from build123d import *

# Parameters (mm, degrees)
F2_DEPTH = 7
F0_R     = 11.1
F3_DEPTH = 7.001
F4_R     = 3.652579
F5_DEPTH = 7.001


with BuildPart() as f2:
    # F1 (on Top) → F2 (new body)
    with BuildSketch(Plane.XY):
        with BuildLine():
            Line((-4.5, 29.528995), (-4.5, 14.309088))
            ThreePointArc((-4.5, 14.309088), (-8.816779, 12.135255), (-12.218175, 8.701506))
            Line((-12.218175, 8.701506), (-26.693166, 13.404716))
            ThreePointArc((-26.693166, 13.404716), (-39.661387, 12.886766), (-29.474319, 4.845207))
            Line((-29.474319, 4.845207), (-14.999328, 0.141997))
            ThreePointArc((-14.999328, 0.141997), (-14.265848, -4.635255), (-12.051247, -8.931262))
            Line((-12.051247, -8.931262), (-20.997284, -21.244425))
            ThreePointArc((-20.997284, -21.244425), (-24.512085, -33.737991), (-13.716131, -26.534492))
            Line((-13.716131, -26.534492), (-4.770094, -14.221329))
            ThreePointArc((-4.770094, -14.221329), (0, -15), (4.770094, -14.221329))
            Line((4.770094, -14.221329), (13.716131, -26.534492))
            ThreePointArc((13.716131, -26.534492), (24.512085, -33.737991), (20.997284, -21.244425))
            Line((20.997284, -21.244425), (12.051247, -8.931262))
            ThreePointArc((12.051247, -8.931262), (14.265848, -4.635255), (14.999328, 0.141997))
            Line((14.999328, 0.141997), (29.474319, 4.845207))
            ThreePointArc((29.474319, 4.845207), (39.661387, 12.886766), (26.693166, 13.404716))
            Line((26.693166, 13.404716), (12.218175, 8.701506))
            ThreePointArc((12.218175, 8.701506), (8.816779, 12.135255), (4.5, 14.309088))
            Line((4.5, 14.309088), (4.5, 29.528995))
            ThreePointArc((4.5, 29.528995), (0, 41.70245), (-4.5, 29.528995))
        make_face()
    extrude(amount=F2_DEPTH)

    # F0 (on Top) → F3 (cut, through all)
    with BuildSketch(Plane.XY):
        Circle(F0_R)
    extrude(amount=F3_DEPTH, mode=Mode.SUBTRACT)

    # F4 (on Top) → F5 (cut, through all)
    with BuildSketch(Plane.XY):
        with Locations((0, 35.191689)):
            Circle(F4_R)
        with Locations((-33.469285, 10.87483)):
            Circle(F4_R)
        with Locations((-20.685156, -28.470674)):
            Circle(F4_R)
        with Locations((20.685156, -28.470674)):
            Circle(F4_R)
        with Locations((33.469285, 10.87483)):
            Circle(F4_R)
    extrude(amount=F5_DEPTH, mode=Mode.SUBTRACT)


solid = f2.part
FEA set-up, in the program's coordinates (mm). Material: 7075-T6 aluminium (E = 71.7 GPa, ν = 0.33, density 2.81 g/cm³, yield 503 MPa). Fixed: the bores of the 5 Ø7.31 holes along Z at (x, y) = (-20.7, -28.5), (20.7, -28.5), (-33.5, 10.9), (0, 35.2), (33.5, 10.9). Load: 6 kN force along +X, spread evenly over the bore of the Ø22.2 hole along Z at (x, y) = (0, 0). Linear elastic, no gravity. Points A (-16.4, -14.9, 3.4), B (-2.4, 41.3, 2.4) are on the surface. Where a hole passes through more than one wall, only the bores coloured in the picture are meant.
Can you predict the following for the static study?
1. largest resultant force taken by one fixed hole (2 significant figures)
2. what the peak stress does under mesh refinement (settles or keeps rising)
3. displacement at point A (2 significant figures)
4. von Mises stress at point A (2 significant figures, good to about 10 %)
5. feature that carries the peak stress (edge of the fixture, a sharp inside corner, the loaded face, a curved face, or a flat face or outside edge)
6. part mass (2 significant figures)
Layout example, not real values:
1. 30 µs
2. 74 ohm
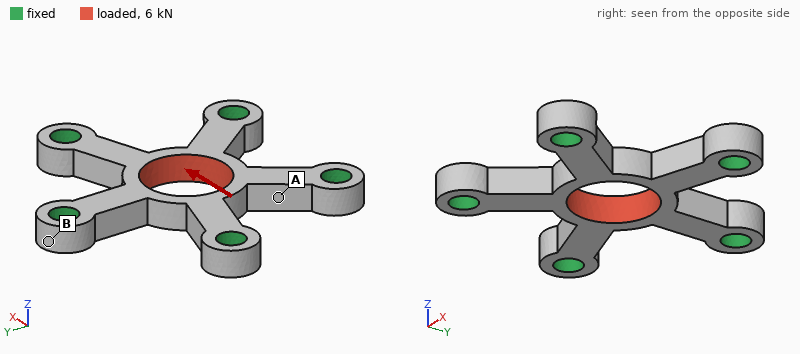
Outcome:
1. 2.1 kN
2. keeps rising
3. 8.3 µm
4. 30 MPa
5. a sharp inside corner
6. 29 g
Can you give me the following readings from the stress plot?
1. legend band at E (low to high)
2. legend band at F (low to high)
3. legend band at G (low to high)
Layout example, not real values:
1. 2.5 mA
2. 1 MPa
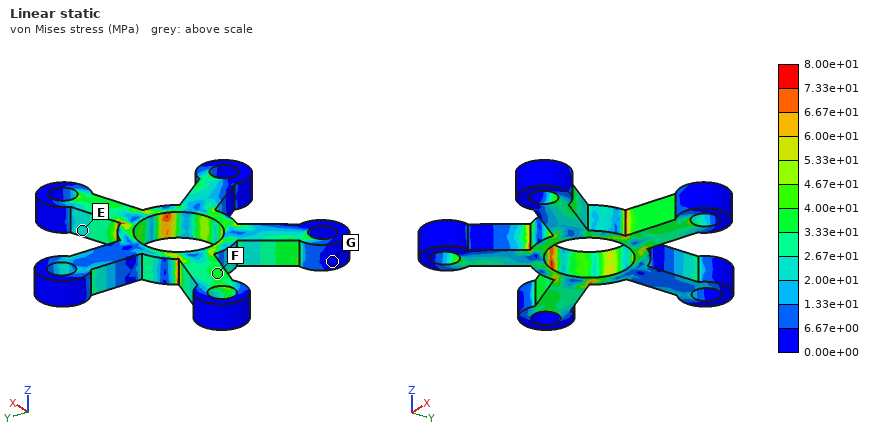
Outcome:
1. 2.00e+01 to 2.67e+01 MPa
2. 3.33e+01 to 4.00e+01 MPa
3. 0.00e+00 to 6.67e+00 MPa
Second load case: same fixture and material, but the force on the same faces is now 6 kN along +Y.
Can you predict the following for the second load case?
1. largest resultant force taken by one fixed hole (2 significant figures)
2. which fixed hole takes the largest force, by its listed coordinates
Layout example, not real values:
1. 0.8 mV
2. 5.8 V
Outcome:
1. 2.2 kN
2. (0, 35.2)
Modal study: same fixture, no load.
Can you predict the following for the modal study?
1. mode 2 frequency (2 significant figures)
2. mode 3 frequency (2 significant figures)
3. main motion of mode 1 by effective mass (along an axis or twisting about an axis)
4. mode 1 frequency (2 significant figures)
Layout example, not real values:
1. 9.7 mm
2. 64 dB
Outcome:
1. 18 kHz
2. 18 kHz
3. along Z
4. 12 kHz
